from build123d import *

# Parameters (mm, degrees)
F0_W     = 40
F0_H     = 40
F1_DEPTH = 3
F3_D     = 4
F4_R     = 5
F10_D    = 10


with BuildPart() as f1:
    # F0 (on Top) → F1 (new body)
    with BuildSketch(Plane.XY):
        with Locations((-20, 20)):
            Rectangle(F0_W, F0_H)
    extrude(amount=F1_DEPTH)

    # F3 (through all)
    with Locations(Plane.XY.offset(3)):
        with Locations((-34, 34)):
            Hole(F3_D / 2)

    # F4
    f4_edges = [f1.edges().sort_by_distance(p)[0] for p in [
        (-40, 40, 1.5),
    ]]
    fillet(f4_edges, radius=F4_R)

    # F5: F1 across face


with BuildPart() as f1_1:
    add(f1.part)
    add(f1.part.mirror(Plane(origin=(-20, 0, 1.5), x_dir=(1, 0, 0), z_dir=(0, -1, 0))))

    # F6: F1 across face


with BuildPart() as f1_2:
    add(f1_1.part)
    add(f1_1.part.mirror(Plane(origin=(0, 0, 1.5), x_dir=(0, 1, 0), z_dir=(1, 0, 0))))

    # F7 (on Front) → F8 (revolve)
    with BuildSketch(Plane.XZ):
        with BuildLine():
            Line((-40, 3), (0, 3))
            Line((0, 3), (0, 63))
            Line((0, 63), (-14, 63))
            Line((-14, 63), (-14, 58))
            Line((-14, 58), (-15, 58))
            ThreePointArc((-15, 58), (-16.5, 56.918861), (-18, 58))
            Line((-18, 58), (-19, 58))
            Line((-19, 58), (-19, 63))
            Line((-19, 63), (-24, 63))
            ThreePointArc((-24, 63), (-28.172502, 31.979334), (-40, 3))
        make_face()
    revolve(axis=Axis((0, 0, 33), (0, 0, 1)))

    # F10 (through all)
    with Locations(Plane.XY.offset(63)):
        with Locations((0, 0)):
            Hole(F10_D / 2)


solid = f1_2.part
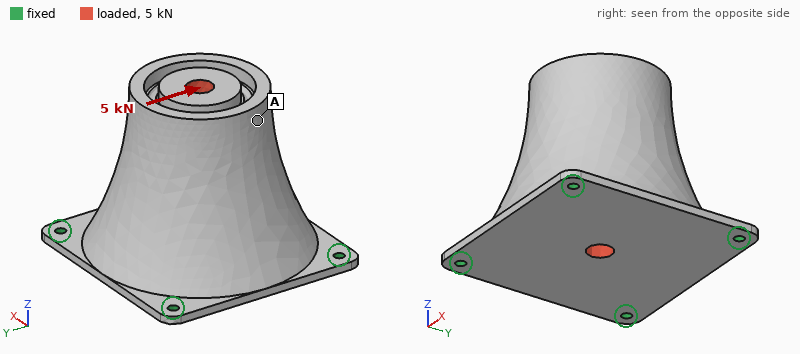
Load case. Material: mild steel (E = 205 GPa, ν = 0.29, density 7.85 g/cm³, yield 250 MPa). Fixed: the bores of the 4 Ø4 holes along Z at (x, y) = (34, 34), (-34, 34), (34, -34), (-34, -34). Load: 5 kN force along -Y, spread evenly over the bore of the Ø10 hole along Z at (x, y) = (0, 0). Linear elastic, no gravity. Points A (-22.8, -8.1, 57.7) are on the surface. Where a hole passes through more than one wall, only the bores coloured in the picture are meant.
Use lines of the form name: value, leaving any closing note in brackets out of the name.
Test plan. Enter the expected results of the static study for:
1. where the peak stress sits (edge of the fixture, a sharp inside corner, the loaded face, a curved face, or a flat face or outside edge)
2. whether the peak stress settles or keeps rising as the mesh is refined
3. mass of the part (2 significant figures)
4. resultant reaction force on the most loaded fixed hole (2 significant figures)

where the peak stress sits: edge of the fixture
whether the peak stress settles or keeps rising as the mesh is refined: keeps rising
mass of the part: 1.4 kg
resultant reaction force on the most loaded fixed hole: 1.9 kN
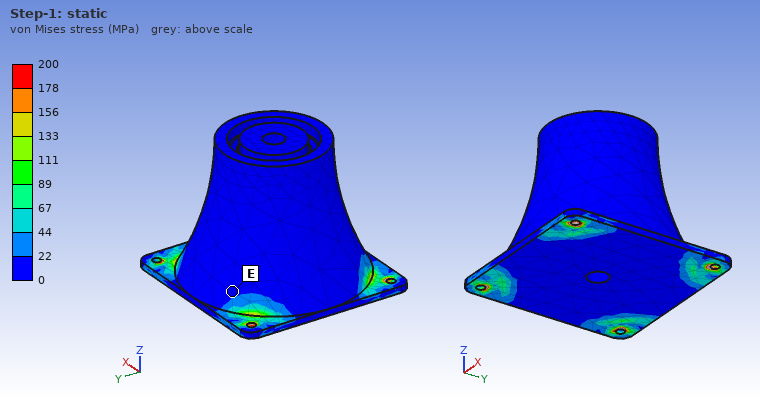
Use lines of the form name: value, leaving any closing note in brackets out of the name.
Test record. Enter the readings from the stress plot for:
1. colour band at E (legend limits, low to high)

colour band at E: 0 to 22 MPa
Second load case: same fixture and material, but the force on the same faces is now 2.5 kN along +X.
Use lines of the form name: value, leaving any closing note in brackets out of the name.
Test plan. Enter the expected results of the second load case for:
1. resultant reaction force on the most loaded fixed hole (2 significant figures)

resultant reaction force on the most loaded fixed hole: 950 N
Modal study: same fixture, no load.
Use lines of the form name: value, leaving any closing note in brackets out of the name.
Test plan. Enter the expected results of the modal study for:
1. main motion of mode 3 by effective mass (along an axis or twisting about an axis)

main motion of mode 3 by effective mass: along Z
